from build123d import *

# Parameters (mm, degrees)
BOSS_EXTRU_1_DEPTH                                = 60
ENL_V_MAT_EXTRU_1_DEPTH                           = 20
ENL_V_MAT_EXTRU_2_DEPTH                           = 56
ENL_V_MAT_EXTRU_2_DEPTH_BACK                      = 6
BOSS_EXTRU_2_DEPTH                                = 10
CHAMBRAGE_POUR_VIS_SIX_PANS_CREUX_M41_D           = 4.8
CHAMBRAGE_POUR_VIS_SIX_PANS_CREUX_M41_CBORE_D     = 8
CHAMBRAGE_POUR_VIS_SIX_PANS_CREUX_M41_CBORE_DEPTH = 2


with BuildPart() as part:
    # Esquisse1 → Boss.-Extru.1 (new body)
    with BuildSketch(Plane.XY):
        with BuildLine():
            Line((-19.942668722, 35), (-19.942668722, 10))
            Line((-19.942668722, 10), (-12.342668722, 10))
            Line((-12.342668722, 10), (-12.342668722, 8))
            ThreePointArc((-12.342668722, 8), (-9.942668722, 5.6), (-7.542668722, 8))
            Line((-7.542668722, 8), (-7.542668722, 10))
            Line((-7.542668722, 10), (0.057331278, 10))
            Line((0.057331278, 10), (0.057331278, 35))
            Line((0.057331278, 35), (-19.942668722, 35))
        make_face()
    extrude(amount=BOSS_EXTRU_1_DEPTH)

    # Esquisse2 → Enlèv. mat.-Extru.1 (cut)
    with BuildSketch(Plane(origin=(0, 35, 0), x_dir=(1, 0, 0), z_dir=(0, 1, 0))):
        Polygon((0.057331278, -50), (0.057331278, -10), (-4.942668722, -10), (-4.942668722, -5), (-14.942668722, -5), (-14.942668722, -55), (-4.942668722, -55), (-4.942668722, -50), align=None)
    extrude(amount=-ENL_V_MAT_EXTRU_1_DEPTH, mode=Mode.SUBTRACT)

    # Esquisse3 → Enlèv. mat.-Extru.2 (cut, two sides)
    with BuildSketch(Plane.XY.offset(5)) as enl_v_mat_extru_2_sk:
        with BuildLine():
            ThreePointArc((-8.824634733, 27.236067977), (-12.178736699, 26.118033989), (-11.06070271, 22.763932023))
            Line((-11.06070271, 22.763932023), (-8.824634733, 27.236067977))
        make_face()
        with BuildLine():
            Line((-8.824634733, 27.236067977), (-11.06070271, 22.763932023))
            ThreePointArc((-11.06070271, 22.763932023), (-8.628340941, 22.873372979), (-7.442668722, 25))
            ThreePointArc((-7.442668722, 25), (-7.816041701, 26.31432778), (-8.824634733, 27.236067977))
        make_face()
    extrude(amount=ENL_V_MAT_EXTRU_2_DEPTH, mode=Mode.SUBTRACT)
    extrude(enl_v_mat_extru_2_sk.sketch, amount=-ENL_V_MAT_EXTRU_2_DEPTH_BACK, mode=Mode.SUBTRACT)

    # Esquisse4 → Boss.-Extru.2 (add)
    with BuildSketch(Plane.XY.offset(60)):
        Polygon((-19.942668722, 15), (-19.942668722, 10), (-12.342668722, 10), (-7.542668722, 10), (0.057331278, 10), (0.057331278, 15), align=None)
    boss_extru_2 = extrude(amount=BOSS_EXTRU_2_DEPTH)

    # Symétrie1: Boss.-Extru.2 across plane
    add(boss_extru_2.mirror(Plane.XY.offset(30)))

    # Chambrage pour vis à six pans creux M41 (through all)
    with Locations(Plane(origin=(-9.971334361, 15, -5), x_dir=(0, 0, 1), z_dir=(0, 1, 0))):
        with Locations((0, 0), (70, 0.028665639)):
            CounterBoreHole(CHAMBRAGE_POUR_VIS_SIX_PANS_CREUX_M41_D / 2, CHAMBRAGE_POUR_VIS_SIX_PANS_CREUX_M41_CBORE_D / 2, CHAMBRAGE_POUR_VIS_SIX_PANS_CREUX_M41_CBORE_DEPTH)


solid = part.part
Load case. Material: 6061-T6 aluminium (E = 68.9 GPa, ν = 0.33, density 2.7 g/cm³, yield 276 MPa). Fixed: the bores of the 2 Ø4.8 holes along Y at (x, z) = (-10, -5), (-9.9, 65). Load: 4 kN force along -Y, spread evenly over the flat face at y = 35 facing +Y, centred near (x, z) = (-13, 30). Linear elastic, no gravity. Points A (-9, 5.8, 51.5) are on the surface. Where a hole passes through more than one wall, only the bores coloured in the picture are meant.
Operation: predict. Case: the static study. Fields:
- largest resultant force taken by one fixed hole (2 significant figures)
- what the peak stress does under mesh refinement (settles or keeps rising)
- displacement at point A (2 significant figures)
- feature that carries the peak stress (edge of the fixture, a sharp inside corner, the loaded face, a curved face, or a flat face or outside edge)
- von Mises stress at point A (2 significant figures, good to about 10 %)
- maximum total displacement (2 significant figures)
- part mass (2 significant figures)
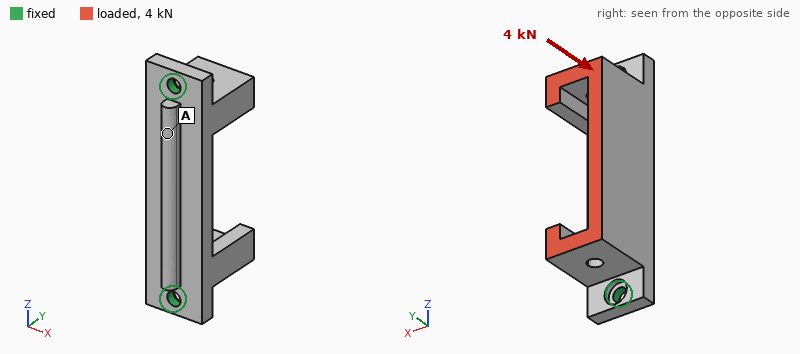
2.2 kN
keeps rising
0.025 mm
edge of the fixture
25 MPa
0.11 mm
50 g
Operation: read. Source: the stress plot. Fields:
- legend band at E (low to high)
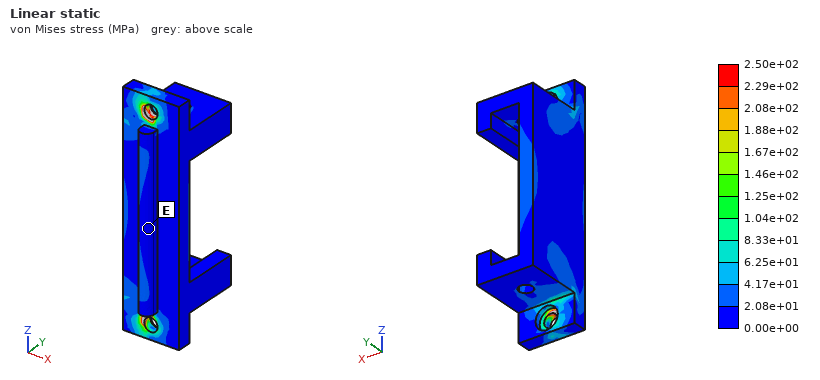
0.00e+00 to 2.08e+01 MPa
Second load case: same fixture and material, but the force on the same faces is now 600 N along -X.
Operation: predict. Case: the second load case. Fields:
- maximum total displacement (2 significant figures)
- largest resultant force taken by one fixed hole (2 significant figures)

0.12 mm
300 N
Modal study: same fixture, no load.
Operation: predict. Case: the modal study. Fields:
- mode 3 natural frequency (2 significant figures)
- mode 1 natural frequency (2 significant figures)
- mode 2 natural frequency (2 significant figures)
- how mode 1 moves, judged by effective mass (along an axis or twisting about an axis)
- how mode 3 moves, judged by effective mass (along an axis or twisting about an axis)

7200 Hz
3400 Hz
6500 Hz
along X
along Y
